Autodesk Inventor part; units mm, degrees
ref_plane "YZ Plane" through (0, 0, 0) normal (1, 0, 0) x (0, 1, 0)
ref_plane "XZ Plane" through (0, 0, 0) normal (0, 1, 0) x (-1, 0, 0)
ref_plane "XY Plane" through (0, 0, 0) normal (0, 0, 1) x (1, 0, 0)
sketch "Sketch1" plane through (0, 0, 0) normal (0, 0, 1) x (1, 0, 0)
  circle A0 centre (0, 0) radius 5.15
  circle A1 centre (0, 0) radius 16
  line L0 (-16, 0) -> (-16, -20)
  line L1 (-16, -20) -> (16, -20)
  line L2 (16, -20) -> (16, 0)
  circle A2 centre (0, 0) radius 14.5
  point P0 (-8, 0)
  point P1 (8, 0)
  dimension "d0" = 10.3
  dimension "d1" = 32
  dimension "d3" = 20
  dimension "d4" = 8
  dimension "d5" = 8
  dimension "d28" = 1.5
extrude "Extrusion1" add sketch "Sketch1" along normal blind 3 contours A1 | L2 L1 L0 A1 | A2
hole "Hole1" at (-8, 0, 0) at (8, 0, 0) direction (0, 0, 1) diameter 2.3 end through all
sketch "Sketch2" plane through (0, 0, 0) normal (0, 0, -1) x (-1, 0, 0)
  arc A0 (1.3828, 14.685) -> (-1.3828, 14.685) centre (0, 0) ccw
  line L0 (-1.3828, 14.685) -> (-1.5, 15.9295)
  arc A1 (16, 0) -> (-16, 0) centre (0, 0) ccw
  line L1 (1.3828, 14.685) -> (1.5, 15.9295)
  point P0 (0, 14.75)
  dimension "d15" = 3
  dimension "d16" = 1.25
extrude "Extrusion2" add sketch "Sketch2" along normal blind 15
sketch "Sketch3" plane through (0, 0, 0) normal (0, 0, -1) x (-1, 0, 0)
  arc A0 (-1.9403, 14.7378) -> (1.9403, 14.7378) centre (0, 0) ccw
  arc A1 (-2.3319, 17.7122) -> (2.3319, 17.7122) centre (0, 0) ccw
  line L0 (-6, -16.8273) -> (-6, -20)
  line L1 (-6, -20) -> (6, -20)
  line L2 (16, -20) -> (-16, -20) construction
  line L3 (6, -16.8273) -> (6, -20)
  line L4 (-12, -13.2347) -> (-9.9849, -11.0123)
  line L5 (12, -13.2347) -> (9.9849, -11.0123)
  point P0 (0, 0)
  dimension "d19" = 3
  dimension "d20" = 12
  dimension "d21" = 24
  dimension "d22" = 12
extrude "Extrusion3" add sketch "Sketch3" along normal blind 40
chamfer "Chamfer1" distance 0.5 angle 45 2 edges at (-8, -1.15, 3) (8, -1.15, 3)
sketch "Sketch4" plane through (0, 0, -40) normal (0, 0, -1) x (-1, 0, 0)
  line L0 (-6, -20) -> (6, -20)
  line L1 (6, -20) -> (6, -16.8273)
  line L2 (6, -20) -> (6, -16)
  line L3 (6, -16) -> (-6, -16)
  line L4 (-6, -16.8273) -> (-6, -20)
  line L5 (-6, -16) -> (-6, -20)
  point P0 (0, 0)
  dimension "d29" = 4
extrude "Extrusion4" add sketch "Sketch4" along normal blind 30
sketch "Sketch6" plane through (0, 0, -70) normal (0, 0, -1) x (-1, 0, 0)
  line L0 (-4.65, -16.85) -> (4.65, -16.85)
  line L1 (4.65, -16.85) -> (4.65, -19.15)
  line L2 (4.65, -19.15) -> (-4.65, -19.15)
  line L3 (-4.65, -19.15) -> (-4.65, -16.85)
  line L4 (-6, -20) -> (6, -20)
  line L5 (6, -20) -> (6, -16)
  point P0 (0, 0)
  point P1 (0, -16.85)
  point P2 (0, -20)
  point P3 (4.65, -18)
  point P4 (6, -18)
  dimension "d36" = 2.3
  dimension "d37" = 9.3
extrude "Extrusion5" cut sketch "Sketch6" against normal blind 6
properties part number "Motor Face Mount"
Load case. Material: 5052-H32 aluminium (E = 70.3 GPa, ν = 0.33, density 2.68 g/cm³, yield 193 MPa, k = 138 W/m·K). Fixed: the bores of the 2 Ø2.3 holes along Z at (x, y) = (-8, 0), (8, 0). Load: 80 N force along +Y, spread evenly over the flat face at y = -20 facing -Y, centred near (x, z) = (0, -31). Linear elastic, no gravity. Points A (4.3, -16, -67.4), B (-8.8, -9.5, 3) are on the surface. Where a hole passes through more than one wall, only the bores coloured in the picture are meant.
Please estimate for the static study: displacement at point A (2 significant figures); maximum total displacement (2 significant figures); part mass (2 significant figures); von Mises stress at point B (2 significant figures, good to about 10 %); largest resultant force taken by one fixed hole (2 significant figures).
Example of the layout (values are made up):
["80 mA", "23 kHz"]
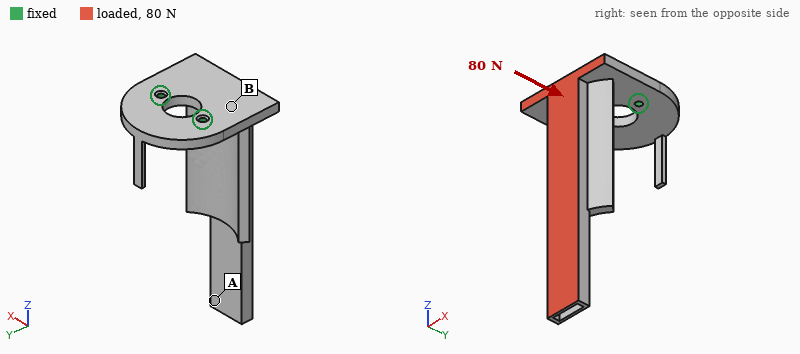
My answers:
["0.81 mm", "0.85 mm", "22 g", "54 MPa", "42 N"]
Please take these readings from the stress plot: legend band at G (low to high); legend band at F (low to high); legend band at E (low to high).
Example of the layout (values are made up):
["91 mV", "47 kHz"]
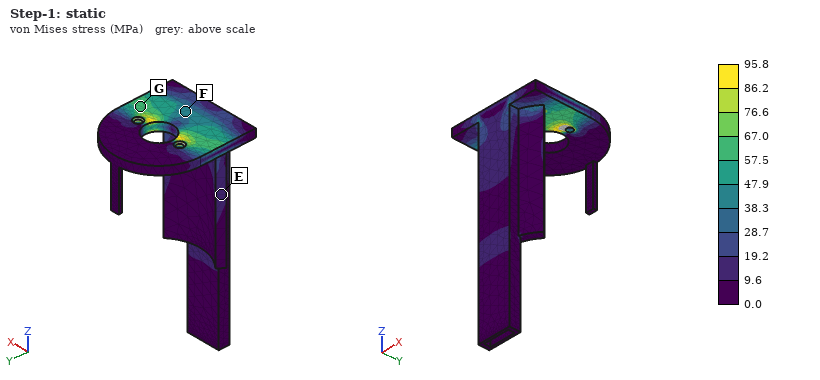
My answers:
["57.5 to 67.0 MPa", "38.3 to 47.9 MPa", "9.6 to 19.2 MPa"]
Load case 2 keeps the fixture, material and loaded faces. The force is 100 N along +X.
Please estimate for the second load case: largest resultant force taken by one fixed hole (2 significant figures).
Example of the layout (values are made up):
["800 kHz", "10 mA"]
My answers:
["190 N"]
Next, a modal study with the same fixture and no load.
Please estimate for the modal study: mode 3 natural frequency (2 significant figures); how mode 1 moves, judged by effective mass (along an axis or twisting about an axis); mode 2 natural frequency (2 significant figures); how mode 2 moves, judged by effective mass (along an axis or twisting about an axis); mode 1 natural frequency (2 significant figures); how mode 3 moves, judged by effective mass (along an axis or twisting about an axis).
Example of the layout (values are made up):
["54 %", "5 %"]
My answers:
["3300 Hz", "along Y", "1300 Hz", "along X", "560 Hz", "along Z"]
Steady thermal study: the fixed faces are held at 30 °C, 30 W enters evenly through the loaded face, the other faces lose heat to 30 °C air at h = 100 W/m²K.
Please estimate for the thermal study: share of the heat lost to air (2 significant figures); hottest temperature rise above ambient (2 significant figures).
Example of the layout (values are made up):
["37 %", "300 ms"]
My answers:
["50 %", "69 K"]
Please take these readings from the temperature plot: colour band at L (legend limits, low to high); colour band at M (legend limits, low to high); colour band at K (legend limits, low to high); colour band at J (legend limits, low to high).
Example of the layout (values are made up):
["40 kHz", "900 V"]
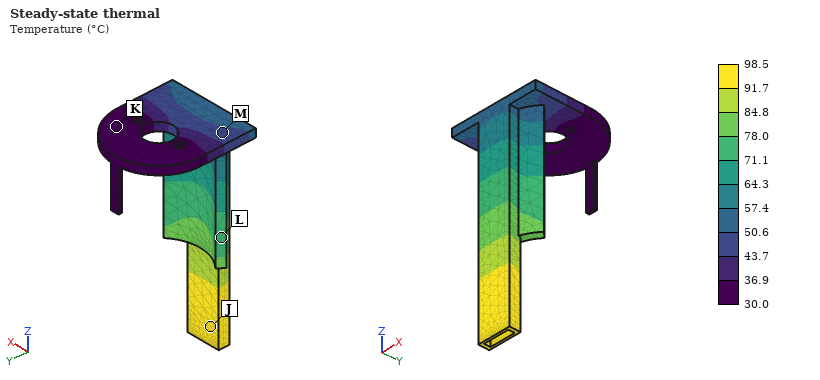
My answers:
["71.1 to 78.0 °C", "43.7 to 50.6 °C", "30.0 to 36.9 °C", "91.7 to 98.5 °C"]
